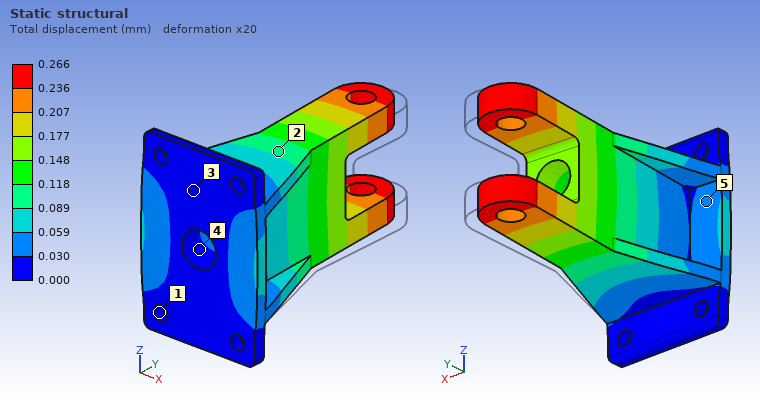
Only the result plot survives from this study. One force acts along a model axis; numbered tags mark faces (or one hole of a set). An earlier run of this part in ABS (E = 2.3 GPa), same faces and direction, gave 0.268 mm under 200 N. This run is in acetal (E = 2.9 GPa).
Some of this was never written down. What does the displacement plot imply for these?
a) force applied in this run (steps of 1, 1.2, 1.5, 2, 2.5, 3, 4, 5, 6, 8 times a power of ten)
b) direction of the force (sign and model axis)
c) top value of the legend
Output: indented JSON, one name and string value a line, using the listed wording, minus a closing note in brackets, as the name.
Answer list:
{
  "force applied in this run": "250 N",
  "direction of the force": "-X",
  "top value of the legend": "0.266 mm"
}
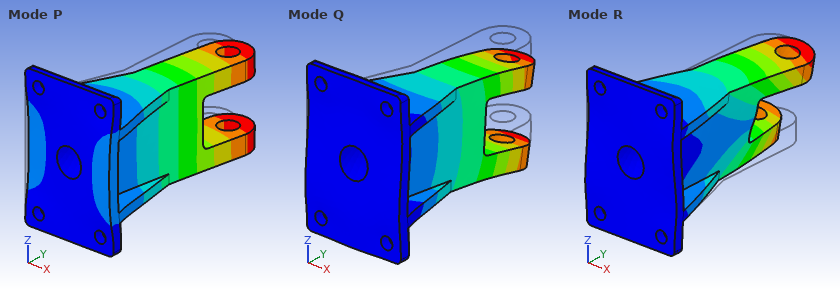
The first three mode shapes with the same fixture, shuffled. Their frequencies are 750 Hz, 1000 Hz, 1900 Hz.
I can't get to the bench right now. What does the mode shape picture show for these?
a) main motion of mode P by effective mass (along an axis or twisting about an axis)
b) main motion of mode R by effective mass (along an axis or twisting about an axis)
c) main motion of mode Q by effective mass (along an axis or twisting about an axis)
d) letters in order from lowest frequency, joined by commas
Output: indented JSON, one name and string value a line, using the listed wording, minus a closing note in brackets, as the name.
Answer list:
{
  "main motion of mode P by effective mass": "along X",
  "main motion of mode R by effective mass": "twisting about Y",
  "main motion of mode Q by effective mass": "along Z",
  "letters in order from lowest frequency, joined by commas": "P, Q, R"
}
